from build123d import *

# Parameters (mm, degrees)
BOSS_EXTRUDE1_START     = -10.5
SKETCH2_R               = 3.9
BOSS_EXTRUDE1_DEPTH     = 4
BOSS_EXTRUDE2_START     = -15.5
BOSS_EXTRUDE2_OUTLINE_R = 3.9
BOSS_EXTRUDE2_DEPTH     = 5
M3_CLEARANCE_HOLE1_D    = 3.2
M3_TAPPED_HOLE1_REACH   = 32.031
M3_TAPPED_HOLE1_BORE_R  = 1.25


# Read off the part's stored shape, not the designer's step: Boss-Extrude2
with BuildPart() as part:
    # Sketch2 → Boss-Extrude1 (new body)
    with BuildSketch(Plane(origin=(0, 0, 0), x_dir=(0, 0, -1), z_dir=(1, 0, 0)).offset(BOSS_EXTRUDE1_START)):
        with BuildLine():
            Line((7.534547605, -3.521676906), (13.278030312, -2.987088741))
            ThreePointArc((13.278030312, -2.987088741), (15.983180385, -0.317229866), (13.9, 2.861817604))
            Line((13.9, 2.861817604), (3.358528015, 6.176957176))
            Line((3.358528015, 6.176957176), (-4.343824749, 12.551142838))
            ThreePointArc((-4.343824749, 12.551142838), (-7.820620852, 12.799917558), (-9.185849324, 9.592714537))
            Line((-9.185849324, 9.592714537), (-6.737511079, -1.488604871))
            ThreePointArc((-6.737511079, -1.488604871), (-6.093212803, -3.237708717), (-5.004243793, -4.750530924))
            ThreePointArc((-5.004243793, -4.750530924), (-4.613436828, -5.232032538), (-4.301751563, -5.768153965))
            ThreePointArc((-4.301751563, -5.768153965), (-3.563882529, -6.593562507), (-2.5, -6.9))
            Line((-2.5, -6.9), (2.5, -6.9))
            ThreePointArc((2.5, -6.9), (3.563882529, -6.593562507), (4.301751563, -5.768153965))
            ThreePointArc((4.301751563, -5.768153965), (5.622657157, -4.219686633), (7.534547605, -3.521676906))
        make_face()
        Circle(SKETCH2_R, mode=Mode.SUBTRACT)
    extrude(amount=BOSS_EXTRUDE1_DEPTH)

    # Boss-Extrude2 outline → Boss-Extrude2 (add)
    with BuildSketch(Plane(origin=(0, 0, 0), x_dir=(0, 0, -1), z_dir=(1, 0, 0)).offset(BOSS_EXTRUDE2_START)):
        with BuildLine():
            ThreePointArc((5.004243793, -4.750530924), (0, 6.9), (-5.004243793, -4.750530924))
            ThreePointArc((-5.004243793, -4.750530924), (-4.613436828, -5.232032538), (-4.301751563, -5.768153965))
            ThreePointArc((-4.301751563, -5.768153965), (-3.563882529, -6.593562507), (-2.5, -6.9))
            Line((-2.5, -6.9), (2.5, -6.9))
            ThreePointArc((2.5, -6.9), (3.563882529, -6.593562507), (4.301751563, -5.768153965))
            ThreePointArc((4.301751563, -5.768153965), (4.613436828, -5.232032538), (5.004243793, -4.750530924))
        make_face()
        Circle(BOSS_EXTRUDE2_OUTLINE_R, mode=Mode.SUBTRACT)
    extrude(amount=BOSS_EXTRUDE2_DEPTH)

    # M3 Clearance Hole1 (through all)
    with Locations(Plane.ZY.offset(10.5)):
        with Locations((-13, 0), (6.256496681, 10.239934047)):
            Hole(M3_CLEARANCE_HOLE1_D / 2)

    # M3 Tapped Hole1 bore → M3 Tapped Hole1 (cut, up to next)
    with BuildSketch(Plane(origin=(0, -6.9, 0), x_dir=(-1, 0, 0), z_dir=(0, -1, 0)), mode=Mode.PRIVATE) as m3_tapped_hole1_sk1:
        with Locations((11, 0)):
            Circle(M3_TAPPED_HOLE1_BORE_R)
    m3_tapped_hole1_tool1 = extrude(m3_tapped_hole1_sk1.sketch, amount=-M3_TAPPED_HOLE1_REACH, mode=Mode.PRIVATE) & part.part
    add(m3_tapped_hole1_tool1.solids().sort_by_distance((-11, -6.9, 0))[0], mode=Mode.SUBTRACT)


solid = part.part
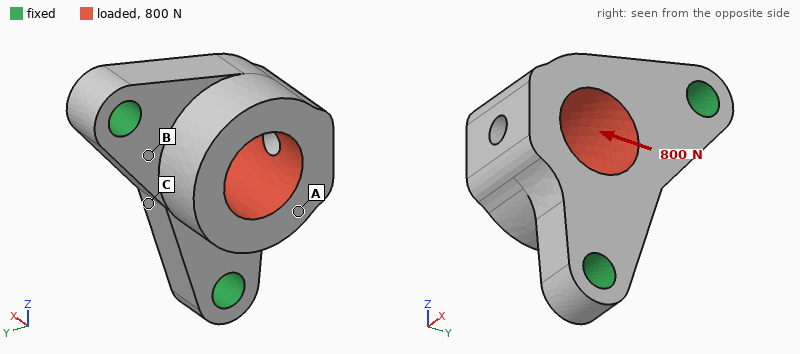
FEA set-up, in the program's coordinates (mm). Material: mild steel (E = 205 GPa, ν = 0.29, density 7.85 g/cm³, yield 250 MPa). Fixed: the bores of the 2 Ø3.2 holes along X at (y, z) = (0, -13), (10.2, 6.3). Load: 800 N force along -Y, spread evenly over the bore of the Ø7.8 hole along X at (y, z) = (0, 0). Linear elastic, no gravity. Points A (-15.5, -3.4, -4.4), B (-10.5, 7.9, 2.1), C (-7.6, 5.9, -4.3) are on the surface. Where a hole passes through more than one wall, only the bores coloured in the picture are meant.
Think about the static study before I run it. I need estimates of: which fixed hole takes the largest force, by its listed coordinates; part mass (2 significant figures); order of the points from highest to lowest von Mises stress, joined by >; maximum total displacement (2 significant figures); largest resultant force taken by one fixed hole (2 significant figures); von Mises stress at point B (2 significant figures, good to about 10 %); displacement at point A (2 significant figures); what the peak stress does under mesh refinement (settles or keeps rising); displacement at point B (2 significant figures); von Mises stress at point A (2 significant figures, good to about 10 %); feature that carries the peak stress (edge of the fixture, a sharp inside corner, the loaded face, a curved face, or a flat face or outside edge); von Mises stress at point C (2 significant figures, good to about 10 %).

(10.2, 6.3)
11 g
B > C > A
9.9 µm
580 N
50 MPa
6.9 µm
keeps rising
1.5 µm
8.9 MPa
edge of the fixture
24 MPa
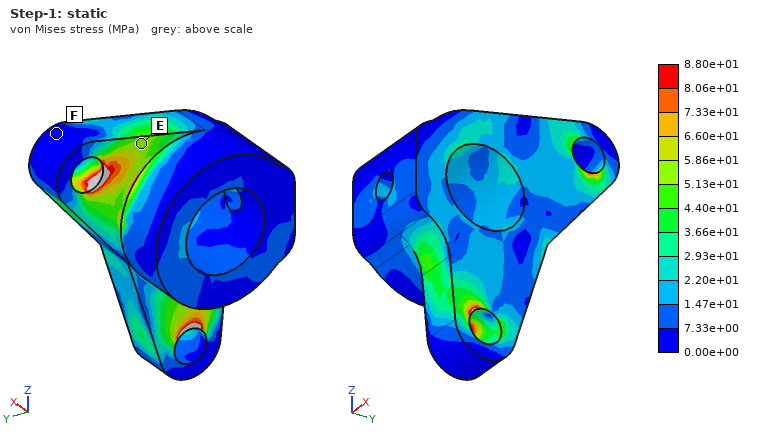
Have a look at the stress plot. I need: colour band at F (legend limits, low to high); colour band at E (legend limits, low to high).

0.00e+00 to 7.33e+00 MPa
5.13e+01 to 5.86e+01 MPa
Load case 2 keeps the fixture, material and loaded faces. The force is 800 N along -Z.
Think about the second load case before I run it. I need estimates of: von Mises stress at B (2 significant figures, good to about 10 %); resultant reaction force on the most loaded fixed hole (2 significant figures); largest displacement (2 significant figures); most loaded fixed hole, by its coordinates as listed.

30 MPa
560 N
5.4 µm
(0, -13)
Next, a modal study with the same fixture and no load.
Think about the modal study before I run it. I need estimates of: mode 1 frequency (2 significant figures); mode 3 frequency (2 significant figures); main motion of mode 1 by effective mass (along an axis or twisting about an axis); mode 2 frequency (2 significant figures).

13 kHz
39 kHz
along X
35 kHz
